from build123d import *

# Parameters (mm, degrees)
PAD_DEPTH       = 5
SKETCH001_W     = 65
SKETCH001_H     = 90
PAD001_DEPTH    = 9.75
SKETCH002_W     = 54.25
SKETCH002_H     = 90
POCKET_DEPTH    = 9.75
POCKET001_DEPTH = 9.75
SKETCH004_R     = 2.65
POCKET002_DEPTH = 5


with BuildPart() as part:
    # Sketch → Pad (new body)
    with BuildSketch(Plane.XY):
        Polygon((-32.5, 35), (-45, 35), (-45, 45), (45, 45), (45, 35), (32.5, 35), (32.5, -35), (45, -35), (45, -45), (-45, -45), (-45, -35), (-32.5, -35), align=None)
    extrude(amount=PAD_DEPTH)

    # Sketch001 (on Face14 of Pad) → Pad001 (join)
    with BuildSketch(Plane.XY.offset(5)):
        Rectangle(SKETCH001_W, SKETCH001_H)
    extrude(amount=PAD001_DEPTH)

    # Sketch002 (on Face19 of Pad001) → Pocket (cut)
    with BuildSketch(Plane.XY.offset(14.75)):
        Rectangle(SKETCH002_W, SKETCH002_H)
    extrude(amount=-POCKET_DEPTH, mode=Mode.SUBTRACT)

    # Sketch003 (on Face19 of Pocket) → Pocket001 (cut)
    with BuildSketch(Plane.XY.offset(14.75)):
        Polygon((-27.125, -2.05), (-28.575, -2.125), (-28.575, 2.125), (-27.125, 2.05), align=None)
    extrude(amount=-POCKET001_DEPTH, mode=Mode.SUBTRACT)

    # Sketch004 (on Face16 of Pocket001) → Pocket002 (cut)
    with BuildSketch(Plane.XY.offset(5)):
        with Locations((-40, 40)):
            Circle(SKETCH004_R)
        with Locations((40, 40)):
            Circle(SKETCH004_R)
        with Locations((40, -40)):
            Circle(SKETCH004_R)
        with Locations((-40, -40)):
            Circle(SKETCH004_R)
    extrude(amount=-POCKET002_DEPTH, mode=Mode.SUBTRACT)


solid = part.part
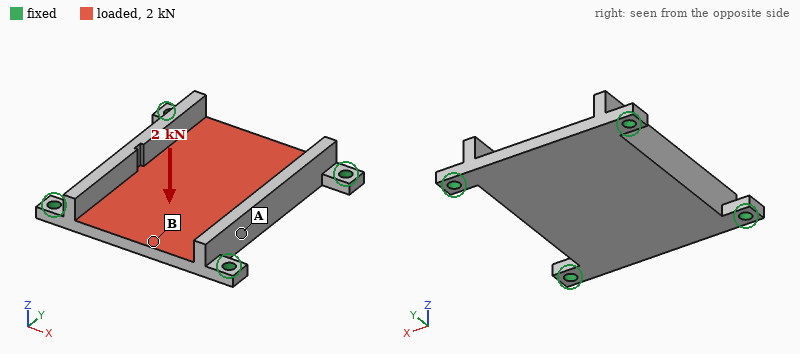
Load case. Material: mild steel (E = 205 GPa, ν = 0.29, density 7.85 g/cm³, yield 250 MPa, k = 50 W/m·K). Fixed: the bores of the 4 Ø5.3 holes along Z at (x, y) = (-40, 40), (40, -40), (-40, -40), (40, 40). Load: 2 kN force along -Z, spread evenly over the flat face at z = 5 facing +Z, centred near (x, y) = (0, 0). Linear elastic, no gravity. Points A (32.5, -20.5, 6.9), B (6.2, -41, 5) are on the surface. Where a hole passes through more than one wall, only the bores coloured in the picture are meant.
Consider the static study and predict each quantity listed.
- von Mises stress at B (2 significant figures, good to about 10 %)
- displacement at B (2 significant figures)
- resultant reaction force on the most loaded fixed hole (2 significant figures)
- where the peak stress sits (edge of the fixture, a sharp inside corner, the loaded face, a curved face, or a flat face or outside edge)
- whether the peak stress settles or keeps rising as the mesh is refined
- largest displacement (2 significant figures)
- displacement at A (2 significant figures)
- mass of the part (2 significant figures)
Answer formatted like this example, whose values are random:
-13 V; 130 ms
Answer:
37 MPa; 32 µm; 520 N; edge of the fixture; keeps rising; 40 µm; 11 µm; 320 g
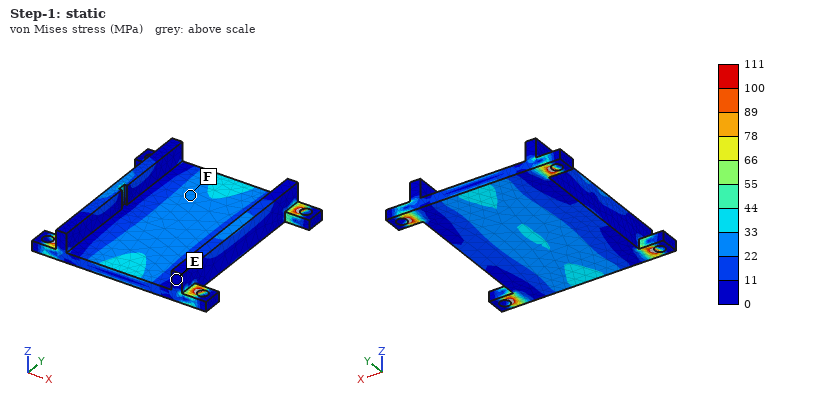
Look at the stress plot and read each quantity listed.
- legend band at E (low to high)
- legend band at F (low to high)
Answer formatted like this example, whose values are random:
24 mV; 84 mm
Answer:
0 to 11 MPa; 22 to 33 MPa
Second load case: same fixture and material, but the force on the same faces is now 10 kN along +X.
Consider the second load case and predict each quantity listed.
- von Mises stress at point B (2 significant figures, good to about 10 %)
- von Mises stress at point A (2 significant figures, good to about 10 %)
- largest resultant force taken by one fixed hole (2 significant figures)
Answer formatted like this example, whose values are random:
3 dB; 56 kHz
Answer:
14 MPa; 11 MPa; 2.6 kN
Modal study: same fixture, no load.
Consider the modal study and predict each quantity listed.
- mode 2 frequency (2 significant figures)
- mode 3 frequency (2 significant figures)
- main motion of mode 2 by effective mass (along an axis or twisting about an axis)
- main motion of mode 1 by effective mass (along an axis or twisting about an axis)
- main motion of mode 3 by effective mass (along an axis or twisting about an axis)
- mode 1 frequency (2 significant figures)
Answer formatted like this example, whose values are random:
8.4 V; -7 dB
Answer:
4500 Hz; 5600 Hz; twisting about X; along Z; twisting about Y; 2700 Hz
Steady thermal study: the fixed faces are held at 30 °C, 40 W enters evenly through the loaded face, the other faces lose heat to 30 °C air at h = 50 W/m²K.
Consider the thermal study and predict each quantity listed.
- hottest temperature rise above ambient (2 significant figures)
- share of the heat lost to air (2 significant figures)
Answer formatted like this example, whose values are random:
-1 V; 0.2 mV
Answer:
38 K; 43 %
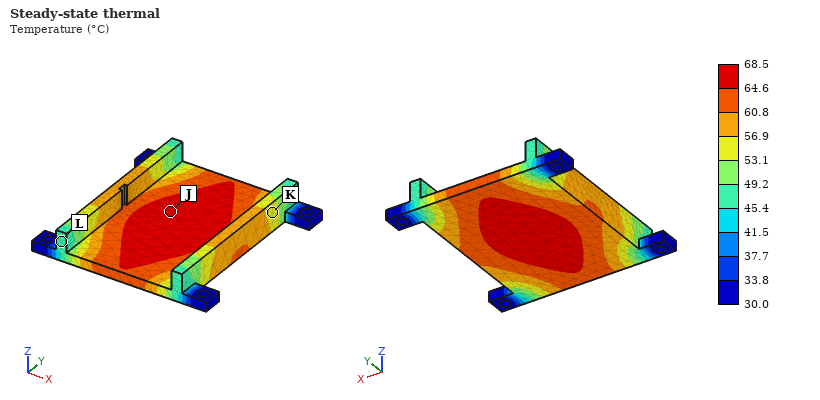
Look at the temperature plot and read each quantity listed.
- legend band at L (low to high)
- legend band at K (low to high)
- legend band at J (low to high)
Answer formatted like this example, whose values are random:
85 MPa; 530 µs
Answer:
45.4 to 49.2 °C; 53.1 to 56.9 °C; 64.6 to 68.5 °C
